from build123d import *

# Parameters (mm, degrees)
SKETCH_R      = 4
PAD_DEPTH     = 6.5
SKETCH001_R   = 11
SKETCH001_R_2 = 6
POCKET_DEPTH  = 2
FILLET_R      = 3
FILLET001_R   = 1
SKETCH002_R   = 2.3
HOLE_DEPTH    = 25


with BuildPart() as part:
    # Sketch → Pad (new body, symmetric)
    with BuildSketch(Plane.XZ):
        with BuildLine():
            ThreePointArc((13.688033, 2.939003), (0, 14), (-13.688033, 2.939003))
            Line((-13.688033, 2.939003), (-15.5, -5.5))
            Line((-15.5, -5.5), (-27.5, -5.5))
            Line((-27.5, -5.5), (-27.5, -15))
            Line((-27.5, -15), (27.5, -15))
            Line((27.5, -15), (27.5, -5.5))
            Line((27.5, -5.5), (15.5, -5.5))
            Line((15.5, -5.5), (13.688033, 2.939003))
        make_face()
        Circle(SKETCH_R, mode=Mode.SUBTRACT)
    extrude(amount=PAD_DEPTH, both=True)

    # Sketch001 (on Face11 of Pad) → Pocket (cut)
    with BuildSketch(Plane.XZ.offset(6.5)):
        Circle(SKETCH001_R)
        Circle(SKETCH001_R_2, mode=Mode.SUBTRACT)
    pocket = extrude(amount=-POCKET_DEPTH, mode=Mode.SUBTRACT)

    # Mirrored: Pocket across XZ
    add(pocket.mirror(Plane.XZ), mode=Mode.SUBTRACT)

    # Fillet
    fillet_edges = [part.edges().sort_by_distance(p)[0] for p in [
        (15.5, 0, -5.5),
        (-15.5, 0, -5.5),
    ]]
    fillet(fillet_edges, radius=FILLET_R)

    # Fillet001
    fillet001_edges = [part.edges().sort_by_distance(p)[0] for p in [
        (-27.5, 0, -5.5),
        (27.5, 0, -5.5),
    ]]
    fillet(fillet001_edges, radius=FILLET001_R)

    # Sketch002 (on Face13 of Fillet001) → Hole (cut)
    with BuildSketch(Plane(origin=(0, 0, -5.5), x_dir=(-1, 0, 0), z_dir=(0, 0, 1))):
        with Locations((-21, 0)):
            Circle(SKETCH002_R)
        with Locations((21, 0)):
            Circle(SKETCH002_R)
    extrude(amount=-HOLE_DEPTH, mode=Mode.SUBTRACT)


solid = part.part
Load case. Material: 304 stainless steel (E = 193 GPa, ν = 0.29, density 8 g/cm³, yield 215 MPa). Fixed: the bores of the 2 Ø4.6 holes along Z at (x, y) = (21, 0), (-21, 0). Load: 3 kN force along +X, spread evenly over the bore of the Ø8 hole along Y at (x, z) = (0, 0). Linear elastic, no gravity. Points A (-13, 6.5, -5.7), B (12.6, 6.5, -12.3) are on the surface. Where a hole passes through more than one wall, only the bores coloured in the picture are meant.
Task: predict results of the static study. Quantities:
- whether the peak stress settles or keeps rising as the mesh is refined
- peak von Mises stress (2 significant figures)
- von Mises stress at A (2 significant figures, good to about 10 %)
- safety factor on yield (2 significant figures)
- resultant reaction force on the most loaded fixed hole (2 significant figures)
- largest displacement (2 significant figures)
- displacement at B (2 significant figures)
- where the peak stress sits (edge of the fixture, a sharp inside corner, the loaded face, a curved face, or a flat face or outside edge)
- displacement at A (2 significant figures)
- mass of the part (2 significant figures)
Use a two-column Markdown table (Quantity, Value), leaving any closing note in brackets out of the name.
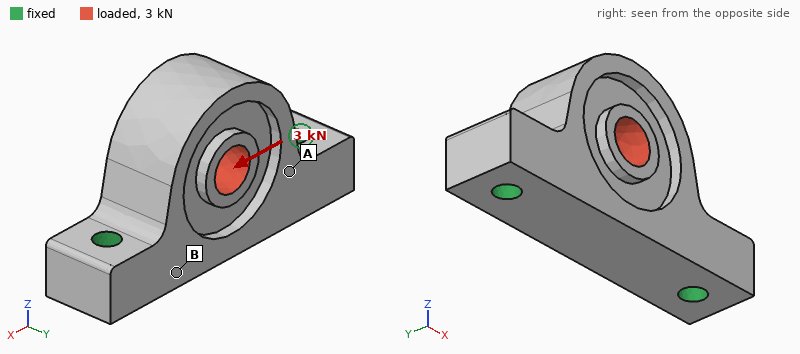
| Quantity | Value |
|---|---|
| whether the peak stress settles or keeps rising as the mesh is refined | settles |
| peak von Mises stress | 59 MPa |
| von Mises stress at A | 6.7 MPa |
| safety factor on yield | 3.6 |
| resultant reaction force on the most loaded fixed hole | 1.7 kN |
| largest displacement | 3.2 µm |
| displacement at B | 0.56 µm |
| where the peak stress sits | a curved face |
| displacement at A | 0.74 µm |
| mass of the part | 87 g |
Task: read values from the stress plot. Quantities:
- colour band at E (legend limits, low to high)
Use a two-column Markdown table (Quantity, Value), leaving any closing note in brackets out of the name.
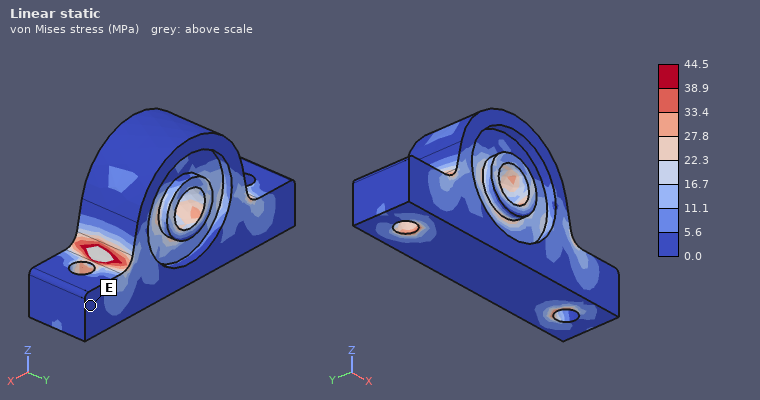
| Quantity | Value |
|---|---|
| colour band at E | 0.0 to 5.6 MPa |
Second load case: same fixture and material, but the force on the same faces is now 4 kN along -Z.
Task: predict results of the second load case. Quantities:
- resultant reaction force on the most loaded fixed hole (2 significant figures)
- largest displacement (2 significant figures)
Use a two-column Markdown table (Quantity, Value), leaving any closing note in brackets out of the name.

| Quantity | Value |
|---|---|
| resultant reaction force on the most loaded fixed hole | 2.1 kN |
| largest displacement | 5.6 µm |
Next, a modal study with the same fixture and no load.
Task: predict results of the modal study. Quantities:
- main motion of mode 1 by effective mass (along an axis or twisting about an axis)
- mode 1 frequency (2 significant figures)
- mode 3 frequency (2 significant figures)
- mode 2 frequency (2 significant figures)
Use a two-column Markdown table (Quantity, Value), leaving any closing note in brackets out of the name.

| Quantity | Value |
|---|---|
| main motion of mode 1 by effective mass | along Y |
| mode 1 frequency | 9000 Hz |
| mode 3 frequency | 22 kHz |
| mode 2 frequency | 21 kHz |
